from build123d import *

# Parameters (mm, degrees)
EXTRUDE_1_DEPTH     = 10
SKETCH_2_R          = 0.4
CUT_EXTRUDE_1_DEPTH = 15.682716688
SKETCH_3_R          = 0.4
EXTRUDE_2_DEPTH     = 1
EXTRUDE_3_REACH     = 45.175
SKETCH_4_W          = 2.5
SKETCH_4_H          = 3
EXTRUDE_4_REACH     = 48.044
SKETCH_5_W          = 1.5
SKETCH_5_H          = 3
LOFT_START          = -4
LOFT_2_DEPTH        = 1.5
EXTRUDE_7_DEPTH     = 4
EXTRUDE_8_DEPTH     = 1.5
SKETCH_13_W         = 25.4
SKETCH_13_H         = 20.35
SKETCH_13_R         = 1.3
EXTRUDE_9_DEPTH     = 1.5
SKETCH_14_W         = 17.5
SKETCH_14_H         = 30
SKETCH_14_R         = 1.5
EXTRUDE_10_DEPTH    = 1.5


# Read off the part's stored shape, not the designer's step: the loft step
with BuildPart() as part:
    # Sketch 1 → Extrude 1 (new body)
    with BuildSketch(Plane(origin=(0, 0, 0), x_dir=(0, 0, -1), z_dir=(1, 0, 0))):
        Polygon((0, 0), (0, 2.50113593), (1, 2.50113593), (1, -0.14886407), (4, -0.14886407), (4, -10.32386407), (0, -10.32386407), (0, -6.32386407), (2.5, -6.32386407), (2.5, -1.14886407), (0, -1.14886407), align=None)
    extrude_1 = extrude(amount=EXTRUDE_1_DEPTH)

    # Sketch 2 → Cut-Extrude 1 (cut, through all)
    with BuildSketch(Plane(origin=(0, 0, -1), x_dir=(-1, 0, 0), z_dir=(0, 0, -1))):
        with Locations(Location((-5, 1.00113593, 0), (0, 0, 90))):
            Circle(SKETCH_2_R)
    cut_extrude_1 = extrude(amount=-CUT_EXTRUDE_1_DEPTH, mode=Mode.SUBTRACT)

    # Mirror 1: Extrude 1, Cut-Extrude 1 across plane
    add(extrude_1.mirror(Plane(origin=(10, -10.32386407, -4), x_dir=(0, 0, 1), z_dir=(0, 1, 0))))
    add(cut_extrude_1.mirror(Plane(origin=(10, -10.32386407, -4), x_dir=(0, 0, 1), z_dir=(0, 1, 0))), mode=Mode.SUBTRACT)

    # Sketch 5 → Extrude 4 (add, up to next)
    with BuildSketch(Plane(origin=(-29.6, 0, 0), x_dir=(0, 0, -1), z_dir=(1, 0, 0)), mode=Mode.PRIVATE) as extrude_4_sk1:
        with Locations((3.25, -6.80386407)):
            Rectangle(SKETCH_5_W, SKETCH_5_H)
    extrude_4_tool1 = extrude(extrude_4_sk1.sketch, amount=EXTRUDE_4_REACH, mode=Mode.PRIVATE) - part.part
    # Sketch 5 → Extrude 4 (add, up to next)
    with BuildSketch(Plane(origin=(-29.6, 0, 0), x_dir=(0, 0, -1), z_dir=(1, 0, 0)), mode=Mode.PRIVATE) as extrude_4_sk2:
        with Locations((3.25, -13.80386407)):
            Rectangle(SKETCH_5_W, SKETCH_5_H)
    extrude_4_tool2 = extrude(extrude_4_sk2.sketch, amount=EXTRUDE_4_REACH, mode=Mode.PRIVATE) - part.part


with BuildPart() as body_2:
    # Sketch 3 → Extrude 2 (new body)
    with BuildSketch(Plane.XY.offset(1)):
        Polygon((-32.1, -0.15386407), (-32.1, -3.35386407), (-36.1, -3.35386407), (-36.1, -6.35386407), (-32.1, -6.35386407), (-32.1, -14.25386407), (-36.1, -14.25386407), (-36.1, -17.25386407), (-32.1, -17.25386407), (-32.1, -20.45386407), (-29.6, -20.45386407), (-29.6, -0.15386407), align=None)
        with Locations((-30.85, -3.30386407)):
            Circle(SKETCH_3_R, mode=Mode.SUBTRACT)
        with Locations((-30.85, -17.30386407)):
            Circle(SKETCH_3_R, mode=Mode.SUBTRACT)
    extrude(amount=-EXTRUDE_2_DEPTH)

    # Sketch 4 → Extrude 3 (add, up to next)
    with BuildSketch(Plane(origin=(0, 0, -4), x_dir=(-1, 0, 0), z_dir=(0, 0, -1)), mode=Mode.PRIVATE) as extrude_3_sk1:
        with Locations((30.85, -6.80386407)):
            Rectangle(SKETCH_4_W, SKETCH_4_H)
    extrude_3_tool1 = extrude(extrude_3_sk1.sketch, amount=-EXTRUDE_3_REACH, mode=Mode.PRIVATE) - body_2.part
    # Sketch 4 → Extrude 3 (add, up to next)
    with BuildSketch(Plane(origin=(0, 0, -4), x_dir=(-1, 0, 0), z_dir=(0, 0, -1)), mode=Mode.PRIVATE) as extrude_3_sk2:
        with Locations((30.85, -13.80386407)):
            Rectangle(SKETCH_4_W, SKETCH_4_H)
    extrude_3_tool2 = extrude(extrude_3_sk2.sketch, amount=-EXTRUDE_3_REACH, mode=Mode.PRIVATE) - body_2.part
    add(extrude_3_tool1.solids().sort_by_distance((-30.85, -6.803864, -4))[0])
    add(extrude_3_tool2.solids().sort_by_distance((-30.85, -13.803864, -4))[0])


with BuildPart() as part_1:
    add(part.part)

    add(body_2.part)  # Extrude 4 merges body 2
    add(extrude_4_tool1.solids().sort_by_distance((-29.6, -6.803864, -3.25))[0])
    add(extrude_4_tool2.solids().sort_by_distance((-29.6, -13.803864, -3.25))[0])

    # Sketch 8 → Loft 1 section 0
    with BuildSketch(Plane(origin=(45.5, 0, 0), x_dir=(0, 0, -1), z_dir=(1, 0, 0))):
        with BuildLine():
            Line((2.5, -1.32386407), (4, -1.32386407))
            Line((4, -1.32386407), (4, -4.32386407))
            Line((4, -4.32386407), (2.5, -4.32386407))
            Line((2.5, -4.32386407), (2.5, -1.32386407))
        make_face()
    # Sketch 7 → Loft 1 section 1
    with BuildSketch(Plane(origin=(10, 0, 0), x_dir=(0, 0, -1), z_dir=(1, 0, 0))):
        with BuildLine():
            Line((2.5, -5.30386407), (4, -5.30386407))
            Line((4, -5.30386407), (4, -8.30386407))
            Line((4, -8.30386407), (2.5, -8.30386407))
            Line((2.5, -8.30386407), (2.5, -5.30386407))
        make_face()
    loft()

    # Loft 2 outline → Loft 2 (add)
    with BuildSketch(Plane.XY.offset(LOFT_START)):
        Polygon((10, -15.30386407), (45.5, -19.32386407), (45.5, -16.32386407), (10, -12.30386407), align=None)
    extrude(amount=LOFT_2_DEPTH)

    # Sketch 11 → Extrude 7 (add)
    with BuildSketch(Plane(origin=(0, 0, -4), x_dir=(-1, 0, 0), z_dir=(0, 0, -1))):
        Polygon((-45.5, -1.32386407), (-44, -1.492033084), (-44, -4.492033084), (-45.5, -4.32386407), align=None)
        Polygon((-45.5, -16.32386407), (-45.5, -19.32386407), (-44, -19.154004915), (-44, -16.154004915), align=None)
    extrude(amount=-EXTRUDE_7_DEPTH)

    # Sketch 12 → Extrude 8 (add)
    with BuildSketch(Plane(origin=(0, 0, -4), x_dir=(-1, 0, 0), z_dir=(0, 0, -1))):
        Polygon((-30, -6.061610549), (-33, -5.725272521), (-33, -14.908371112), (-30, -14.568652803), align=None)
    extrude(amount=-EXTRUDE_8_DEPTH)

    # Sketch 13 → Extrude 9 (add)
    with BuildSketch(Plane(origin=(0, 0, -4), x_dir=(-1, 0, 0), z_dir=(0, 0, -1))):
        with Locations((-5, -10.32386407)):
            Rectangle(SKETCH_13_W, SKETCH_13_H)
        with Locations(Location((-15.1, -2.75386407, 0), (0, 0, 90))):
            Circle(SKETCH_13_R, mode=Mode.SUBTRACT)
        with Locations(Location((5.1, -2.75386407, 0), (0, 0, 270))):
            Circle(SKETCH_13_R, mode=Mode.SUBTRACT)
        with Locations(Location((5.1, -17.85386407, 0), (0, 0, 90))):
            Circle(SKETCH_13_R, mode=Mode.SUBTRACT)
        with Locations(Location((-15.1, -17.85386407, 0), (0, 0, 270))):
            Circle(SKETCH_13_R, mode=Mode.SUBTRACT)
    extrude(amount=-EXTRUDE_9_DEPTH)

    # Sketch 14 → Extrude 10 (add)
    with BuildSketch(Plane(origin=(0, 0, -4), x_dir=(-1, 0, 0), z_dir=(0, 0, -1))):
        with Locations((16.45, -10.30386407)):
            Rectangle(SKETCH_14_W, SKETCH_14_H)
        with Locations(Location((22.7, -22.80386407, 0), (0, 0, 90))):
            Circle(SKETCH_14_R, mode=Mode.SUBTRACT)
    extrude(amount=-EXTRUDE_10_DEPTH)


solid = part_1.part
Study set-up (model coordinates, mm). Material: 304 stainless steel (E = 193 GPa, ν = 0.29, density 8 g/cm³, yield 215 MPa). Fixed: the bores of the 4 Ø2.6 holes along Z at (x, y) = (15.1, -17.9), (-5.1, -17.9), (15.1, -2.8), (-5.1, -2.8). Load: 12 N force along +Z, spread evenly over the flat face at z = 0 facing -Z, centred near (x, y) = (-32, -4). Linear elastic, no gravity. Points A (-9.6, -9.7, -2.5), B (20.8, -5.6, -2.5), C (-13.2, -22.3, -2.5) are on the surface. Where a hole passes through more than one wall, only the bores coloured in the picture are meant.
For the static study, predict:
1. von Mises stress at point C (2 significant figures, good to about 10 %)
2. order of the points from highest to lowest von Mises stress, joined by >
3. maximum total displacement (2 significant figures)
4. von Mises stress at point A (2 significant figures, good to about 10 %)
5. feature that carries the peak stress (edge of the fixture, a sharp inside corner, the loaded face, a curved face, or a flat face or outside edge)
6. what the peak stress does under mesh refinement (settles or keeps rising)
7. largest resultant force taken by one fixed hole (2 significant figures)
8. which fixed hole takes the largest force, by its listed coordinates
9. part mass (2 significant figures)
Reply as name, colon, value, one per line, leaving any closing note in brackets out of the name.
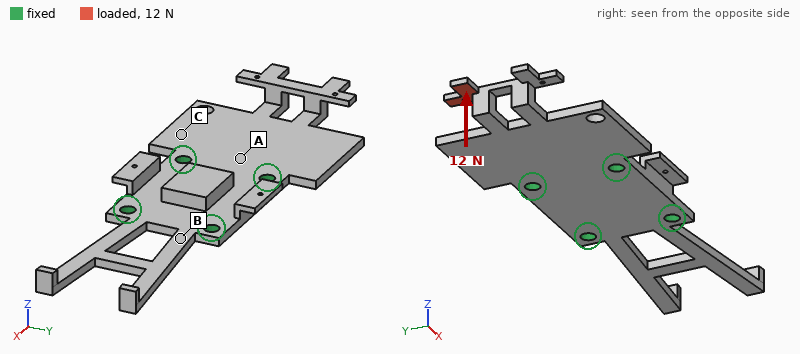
von Mises stress at point C: 16 MPa
order of the points from highest to lowest von Mises stress, joined by >: A > C > B
maximum total displacement: 99 µm
von Mises stress at point A: 27 MPa
feature that carries the peak stress: edge of the fixture
what the peak stress does under mesh refinement: keeps rising
largest resultant force taken by one fixed hole: 12 N
which fixed hole takes the largest force, by its listed coordinates: (-5.1, -2.8)
part mass: 18 g
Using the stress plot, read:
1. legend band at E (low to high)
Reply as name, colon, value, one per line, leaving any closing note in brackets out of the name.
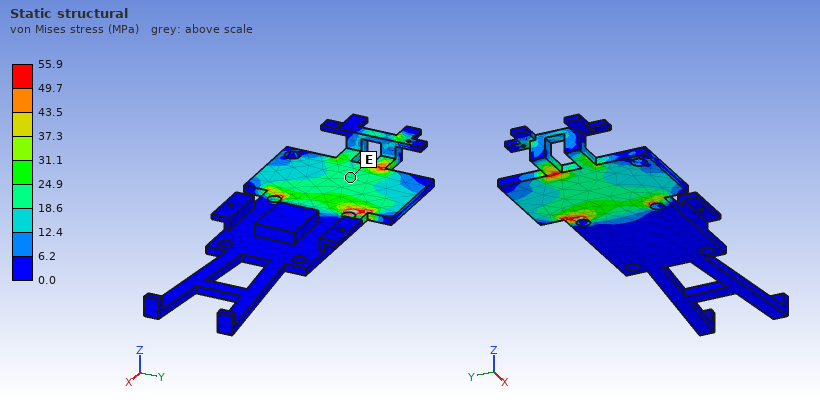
legend band at E: 18.6 to 24.9 MPa
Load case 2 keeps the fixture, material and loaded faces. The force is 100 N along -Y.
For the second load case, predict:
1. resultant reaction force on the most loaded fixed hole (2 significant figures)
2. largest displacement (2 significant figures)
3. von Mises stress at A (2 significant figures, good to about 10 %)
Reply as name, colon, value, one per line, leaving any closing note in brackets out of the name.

resultant reaction force on the most loaded fixed hole: 170 N
largest displacement: 61 µm
von Mises stress at A: 26 MPa
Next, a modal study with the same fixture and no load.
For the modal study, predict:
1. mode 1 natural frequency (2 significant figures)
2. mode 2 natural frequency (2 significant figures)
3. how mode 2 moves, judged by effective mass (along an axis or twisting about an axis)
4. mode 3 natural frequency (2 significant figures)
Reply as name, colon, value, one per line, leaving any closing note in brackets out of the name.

mode 1 natural frequency: 1200 Hz
mode 2 natural frequency: 1700 Hz
how mode 2 moves, judged by effective mass: along Z
mode 3 natural frequency: 2400 Hz
